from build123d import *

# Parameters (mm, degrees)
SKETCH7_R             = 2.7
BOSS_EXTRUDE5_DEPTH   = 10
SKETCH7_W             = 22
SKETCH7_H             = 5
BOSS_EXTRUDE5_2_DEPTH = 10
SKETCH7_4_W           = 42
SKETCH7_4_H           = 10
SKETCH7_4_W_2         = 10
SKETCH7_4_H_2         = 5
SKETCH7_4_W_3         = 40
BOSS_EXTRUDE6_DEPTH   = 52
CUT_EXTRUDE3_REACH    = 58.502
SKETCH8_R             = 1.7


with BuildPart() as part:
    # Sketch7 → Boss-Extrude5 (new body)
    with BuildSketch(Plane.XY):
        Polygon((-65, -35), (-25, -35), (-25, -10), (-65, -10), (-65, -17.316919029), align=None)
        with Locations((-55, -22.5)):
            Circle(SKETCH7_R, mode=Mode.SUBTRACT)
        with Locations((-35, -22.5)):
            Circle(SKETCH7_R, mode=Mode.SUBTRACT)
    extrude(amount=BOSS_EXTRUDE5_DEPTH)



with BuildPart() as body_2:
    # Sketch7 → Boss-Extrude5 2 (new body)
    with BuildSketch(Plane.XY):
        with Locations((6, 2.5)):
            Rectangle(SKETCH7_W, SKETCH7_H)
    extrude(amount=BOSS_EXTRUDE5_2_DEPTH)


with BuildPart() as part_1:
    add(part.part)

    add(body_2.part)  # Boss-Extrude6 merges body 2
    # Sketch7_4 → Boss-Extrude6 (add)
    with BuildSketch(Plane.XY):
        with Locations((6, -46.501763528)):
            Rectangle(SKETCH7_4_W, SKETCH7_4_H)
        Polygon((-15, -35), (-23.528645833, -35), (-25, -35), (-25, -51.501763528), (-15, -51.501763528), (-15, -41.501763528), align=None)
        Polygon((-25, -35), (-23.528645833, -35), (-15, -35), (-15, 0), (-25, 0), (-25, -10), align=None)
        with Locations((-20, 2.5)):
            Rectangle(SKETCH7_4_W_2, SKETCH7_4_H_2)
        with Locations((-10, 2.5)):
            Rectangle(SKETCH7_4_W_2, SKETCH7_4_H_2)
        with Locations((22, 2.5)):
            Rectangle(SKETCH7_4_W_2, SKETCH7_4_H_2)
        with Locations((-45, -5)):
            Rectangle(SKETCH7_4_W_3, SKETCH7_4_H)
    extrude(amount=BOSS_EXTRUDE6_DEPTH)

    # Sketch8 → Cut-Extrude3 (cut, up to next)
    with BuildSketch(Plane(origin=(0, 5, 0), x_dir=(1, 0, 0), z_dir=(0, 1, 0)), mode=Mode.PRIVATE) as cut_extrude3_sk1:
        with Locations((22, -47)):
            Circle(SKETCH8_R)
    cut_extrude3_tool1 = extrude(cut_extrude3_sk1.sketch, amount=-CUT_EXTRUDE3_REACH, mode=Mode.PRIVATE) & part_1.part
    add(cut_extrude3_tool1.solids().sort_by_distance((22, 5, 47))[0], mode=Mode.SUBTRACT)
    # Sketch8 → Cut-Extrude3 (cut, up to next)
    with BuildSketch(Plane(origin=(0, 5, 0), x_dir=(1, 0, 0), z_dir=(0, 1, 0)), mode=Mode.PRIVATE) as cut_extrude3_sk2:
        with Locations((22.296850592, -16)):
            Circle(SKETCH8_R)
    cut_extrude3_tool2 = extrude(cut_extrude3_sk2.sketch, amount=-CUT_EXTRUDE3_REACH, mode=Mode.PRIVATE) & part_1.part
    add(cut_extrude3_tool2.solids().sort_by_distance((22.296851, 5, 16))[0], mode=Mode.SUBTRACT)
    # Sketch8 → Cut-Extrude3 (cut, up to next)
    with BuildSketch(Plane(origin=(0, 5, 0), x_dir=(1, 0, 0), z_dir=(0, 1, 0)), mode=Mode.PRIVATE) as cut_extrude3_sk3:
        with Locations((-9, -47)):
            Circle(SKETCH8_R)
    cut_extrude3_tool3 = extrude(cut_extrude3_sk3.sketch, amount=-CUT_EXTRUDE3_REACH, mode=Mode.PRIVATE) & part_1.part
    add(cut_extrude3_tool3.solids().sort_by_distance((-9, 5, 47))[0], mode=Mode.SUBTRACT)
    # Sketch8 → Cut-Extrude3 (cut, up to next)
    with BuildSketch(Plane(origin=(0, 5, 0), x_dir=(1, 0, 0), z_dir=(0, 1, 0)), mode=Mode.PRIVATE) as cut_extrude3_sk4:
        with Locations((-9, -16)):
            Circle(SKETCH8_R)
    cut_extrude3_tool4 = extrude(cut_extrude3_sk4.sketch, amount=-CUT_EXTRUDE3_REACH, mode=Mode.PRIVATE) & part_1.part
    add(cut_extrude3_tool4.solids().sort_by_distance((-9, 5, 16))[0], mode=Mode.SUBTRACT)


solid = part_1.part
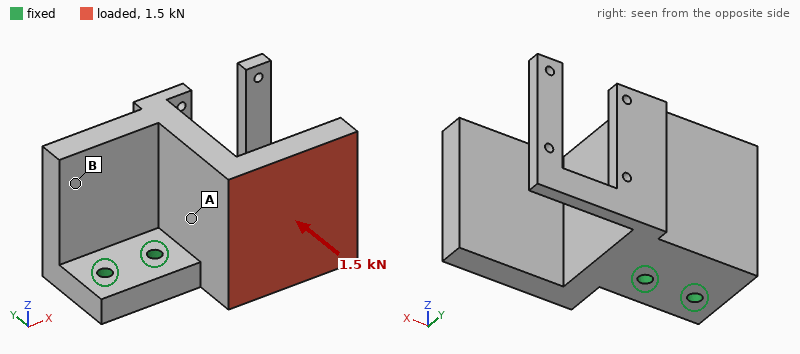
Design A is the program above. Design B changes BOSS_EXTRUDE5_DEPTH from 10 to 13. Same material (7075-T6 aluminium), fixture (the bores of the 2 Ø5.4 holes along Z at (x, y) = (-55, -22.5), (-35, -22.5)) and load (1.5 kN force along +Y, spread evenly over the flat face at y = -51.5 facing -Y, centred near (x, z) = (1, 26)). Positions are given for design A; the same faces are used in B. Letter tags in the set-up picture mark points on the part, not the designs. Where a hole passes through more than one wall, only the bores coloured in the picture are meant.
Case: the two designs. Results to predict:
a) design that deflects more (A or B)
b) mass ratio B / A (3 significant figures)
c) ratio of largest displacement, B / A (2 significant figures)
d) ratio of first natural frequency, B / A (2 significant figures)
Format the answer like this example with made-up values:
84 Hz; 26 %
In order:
A; 1.03; 0.84; 1.0
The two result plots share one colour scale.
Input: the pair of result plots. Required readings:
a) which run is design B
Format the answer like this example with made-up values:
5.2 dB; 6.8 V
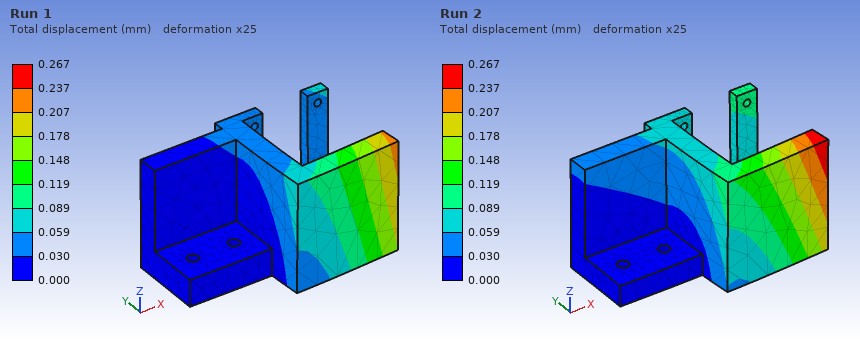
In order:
Run 1
